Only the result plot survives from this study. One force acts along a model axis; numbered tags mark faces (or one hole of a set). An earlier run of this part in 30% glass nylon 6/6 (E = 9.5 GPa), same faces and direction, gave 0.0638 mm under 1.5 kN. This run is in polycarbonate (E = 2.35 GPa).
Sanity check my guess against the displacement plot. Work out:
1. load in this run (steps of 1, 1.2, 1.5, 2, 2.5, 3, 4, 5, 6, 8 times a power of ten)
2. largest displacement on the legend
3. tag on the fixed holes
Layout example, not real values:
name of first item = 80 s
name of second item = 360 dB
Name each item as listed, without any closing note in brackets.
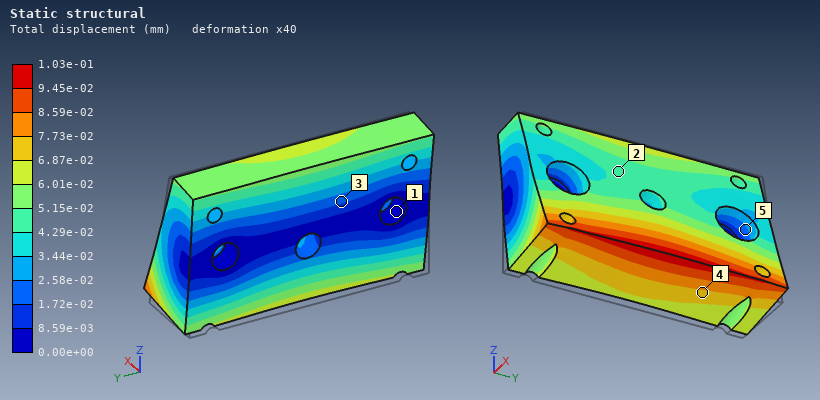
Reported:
load in this run = 600 N
largest displacement on the legend = 1.03e-01 mm
tag on the fixed holes = 1
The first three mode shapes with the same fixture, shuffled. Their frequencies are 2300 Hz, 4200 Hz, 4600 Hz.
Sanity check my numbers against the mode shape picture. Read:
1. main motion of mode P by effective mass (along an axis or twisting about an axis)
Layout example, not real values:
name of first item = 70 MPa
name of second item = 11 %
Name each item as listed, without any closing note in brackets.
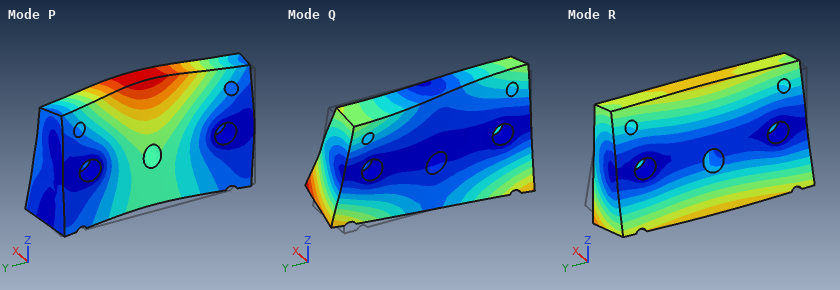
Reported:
main motion of mode P by effective mass = along X
